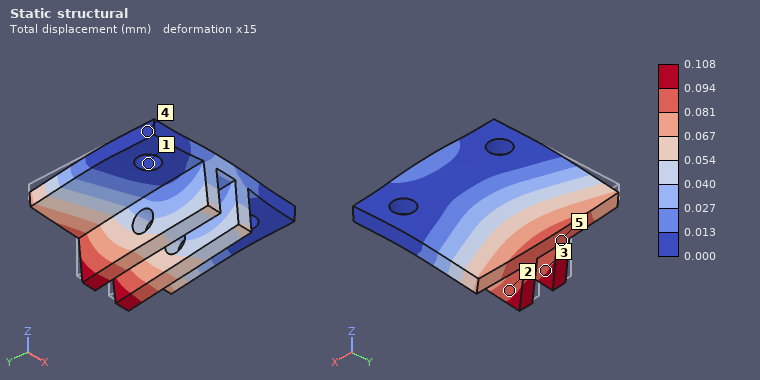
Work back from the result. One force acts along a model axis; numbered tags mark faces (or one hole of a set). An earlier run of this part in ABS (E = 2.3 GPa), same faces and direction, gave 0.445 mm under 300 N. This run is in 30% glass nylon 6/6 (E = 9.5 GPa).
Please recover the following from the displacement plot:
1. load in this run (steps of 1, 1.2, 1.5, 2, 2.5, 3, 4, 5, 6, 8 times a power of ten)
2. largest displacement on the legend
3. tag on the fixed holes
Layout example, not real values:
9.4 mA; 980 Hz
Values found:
300 N; 0.108 mm; 1
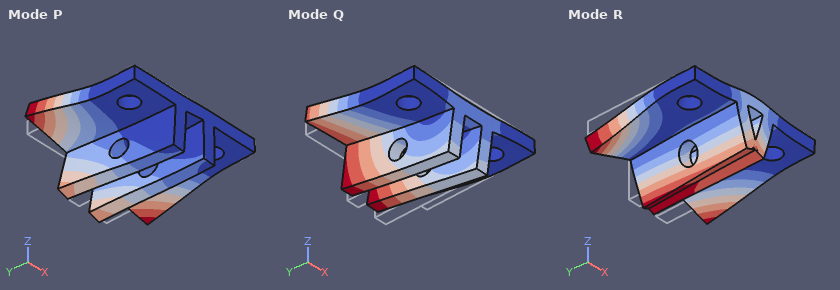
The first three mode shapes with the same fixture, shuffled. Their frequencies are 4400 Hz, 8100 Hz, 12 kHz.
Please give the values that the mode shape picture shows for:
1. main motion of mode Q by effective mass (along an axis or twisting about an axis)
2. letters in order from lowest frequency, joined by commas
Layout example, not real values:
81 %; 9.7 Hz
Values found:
along Z; Q, P, R
